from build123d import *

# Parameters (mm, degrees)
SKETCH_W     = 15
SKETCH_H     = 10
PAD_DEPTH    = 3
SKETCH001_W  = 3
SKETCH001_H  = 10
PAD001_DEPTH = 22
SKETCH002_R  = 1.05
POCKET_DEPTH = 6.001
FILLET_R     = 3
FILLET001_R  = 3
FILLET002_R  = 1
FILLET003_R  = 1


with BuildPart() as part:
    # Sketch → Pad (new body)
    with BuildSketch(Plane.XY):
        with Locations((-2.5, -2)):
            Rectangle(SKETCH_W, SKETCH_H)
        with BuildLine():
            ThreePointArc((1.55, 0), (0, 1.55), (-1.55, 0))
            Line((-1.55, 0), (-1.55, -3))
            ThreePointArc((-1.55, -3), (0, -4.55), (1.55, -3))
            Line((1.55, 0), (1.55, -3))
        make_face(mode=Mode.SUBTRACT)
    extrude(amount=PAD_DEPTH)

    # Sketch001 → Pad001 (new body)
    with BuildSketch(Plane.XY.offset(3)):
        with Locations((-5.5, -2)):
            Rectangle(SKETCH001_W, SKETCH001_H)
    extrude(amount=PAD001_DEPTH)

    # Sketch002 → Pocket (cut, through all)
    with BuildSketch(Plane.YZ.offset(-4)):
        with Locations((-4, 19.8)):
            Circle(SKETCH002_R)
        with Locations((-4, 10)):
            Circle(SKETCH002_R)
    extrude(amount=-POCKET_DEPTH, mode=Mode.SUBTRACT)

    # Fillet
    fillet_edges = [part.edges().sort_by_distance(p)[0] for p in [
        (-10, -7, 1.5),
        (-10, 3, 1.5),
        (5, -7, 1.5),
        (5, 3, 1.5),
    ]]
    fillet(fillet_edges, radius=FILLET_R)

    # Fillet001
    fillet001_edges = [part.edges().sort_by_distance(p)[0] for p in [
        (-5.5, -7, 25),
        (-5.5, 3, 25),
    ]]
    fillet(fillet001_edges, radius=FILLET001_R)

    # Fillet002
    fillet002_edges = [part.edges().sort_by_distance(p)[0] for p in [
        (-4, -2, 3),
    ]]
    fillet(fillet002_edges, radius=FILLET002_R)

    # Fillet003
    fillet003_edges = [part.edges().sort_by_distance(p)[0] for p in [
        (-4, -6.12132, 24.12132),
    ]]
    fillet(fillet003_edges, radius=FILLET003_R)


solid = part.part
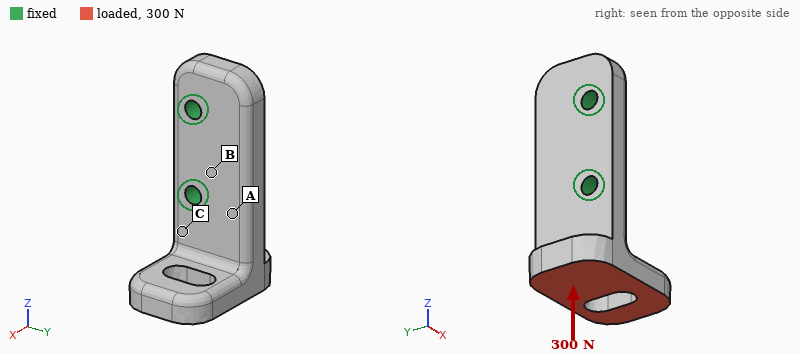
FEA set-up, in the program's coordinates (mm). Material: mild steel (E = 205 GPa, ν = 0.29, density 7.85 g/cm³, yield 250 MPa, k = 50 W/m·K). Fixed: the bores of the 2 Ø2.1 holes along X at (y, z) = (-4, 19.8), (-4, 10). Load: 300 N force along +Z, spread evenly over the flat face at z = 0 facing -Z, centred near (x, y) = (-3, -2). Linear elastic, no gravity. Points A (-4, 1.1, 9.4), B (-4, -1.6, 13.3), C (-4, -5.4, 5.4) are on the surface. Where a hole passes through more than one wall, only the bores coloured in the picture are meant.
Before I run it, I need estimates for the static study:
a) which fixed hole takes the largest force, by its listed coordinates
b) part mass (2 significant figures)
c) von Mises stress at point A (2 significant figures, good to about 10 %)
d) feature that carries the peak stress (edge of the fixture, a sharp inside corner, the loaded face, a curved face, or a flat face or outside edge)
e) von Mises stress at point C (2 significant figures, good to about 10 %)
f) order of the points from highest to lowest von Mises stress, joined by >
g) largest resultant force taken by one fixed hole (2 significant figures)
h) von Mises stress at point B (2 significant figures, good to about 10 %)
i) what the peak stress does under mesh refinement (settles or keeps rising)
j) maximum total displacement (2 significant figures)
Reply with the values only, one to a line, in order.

(-4, 10)
7.8 g
43 MPa
edge of the fixture
68 MPa
C > A > B
250 N
13 MPa
keeps rising
25 µm
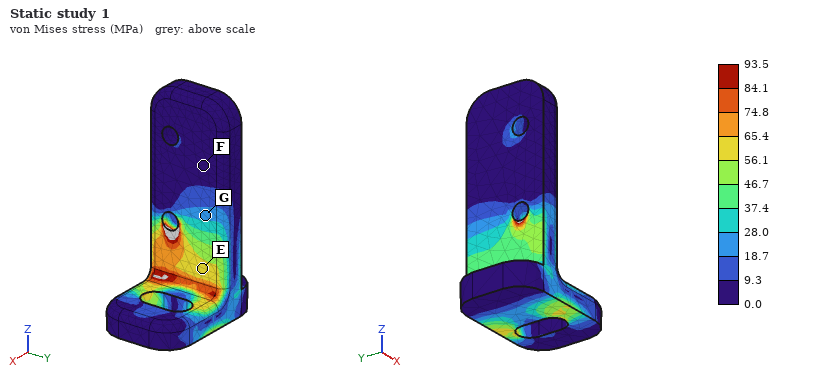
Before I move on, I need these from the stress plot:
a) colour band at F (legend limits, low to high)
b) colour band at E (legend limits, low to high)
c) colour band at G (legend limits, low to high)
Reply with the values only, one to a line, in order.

0.0 to 9.3 MPa
56.1 to 65.4 MPa
18.7 to 28.0 MPa
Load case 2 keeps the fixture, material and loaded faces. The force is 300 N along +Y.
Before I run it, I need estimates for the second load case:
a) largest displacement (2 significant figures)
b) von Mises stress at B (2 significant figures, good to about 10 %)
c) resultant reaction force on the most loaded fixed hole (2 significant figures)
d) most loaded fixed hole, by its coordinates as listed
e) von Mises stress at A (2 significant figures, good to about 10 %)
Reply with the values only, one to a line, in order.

17 µm
12 MPa
530 N
(-4, 10)
33 MPa
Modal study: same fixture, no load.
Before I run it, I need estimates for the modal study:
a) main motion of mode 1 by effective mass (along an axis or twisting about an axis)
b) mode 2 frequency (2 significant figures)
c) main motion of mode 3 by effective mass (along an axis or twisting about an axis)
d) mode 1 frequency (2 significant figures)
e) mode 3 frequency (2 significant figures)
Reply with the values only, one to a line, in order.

along X
13 kHz
along X
9100 Hz
23 kHz
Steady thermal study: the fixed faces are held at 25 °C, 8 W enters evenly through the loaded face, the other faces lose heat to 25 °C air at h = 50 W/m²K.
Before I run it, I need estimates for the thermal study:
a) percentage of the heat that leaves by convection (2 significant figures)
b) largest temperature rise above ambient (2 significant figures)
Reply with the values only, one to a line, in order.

11 %
66 K
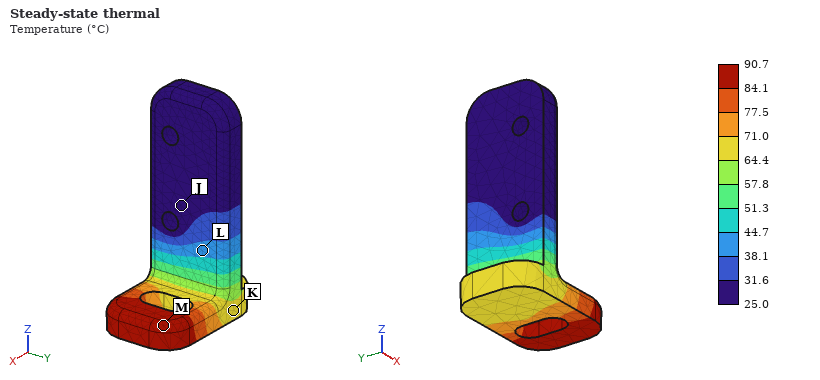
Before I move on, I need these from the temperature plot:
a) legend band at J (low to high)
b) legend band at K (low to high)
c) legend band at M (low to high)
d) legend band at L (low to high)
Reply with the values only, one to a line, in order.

25.0 to 31.6 °C
64.4 to 71.0 °C
84.1 to 90.7 °C
38.1 to 44.7 °C
